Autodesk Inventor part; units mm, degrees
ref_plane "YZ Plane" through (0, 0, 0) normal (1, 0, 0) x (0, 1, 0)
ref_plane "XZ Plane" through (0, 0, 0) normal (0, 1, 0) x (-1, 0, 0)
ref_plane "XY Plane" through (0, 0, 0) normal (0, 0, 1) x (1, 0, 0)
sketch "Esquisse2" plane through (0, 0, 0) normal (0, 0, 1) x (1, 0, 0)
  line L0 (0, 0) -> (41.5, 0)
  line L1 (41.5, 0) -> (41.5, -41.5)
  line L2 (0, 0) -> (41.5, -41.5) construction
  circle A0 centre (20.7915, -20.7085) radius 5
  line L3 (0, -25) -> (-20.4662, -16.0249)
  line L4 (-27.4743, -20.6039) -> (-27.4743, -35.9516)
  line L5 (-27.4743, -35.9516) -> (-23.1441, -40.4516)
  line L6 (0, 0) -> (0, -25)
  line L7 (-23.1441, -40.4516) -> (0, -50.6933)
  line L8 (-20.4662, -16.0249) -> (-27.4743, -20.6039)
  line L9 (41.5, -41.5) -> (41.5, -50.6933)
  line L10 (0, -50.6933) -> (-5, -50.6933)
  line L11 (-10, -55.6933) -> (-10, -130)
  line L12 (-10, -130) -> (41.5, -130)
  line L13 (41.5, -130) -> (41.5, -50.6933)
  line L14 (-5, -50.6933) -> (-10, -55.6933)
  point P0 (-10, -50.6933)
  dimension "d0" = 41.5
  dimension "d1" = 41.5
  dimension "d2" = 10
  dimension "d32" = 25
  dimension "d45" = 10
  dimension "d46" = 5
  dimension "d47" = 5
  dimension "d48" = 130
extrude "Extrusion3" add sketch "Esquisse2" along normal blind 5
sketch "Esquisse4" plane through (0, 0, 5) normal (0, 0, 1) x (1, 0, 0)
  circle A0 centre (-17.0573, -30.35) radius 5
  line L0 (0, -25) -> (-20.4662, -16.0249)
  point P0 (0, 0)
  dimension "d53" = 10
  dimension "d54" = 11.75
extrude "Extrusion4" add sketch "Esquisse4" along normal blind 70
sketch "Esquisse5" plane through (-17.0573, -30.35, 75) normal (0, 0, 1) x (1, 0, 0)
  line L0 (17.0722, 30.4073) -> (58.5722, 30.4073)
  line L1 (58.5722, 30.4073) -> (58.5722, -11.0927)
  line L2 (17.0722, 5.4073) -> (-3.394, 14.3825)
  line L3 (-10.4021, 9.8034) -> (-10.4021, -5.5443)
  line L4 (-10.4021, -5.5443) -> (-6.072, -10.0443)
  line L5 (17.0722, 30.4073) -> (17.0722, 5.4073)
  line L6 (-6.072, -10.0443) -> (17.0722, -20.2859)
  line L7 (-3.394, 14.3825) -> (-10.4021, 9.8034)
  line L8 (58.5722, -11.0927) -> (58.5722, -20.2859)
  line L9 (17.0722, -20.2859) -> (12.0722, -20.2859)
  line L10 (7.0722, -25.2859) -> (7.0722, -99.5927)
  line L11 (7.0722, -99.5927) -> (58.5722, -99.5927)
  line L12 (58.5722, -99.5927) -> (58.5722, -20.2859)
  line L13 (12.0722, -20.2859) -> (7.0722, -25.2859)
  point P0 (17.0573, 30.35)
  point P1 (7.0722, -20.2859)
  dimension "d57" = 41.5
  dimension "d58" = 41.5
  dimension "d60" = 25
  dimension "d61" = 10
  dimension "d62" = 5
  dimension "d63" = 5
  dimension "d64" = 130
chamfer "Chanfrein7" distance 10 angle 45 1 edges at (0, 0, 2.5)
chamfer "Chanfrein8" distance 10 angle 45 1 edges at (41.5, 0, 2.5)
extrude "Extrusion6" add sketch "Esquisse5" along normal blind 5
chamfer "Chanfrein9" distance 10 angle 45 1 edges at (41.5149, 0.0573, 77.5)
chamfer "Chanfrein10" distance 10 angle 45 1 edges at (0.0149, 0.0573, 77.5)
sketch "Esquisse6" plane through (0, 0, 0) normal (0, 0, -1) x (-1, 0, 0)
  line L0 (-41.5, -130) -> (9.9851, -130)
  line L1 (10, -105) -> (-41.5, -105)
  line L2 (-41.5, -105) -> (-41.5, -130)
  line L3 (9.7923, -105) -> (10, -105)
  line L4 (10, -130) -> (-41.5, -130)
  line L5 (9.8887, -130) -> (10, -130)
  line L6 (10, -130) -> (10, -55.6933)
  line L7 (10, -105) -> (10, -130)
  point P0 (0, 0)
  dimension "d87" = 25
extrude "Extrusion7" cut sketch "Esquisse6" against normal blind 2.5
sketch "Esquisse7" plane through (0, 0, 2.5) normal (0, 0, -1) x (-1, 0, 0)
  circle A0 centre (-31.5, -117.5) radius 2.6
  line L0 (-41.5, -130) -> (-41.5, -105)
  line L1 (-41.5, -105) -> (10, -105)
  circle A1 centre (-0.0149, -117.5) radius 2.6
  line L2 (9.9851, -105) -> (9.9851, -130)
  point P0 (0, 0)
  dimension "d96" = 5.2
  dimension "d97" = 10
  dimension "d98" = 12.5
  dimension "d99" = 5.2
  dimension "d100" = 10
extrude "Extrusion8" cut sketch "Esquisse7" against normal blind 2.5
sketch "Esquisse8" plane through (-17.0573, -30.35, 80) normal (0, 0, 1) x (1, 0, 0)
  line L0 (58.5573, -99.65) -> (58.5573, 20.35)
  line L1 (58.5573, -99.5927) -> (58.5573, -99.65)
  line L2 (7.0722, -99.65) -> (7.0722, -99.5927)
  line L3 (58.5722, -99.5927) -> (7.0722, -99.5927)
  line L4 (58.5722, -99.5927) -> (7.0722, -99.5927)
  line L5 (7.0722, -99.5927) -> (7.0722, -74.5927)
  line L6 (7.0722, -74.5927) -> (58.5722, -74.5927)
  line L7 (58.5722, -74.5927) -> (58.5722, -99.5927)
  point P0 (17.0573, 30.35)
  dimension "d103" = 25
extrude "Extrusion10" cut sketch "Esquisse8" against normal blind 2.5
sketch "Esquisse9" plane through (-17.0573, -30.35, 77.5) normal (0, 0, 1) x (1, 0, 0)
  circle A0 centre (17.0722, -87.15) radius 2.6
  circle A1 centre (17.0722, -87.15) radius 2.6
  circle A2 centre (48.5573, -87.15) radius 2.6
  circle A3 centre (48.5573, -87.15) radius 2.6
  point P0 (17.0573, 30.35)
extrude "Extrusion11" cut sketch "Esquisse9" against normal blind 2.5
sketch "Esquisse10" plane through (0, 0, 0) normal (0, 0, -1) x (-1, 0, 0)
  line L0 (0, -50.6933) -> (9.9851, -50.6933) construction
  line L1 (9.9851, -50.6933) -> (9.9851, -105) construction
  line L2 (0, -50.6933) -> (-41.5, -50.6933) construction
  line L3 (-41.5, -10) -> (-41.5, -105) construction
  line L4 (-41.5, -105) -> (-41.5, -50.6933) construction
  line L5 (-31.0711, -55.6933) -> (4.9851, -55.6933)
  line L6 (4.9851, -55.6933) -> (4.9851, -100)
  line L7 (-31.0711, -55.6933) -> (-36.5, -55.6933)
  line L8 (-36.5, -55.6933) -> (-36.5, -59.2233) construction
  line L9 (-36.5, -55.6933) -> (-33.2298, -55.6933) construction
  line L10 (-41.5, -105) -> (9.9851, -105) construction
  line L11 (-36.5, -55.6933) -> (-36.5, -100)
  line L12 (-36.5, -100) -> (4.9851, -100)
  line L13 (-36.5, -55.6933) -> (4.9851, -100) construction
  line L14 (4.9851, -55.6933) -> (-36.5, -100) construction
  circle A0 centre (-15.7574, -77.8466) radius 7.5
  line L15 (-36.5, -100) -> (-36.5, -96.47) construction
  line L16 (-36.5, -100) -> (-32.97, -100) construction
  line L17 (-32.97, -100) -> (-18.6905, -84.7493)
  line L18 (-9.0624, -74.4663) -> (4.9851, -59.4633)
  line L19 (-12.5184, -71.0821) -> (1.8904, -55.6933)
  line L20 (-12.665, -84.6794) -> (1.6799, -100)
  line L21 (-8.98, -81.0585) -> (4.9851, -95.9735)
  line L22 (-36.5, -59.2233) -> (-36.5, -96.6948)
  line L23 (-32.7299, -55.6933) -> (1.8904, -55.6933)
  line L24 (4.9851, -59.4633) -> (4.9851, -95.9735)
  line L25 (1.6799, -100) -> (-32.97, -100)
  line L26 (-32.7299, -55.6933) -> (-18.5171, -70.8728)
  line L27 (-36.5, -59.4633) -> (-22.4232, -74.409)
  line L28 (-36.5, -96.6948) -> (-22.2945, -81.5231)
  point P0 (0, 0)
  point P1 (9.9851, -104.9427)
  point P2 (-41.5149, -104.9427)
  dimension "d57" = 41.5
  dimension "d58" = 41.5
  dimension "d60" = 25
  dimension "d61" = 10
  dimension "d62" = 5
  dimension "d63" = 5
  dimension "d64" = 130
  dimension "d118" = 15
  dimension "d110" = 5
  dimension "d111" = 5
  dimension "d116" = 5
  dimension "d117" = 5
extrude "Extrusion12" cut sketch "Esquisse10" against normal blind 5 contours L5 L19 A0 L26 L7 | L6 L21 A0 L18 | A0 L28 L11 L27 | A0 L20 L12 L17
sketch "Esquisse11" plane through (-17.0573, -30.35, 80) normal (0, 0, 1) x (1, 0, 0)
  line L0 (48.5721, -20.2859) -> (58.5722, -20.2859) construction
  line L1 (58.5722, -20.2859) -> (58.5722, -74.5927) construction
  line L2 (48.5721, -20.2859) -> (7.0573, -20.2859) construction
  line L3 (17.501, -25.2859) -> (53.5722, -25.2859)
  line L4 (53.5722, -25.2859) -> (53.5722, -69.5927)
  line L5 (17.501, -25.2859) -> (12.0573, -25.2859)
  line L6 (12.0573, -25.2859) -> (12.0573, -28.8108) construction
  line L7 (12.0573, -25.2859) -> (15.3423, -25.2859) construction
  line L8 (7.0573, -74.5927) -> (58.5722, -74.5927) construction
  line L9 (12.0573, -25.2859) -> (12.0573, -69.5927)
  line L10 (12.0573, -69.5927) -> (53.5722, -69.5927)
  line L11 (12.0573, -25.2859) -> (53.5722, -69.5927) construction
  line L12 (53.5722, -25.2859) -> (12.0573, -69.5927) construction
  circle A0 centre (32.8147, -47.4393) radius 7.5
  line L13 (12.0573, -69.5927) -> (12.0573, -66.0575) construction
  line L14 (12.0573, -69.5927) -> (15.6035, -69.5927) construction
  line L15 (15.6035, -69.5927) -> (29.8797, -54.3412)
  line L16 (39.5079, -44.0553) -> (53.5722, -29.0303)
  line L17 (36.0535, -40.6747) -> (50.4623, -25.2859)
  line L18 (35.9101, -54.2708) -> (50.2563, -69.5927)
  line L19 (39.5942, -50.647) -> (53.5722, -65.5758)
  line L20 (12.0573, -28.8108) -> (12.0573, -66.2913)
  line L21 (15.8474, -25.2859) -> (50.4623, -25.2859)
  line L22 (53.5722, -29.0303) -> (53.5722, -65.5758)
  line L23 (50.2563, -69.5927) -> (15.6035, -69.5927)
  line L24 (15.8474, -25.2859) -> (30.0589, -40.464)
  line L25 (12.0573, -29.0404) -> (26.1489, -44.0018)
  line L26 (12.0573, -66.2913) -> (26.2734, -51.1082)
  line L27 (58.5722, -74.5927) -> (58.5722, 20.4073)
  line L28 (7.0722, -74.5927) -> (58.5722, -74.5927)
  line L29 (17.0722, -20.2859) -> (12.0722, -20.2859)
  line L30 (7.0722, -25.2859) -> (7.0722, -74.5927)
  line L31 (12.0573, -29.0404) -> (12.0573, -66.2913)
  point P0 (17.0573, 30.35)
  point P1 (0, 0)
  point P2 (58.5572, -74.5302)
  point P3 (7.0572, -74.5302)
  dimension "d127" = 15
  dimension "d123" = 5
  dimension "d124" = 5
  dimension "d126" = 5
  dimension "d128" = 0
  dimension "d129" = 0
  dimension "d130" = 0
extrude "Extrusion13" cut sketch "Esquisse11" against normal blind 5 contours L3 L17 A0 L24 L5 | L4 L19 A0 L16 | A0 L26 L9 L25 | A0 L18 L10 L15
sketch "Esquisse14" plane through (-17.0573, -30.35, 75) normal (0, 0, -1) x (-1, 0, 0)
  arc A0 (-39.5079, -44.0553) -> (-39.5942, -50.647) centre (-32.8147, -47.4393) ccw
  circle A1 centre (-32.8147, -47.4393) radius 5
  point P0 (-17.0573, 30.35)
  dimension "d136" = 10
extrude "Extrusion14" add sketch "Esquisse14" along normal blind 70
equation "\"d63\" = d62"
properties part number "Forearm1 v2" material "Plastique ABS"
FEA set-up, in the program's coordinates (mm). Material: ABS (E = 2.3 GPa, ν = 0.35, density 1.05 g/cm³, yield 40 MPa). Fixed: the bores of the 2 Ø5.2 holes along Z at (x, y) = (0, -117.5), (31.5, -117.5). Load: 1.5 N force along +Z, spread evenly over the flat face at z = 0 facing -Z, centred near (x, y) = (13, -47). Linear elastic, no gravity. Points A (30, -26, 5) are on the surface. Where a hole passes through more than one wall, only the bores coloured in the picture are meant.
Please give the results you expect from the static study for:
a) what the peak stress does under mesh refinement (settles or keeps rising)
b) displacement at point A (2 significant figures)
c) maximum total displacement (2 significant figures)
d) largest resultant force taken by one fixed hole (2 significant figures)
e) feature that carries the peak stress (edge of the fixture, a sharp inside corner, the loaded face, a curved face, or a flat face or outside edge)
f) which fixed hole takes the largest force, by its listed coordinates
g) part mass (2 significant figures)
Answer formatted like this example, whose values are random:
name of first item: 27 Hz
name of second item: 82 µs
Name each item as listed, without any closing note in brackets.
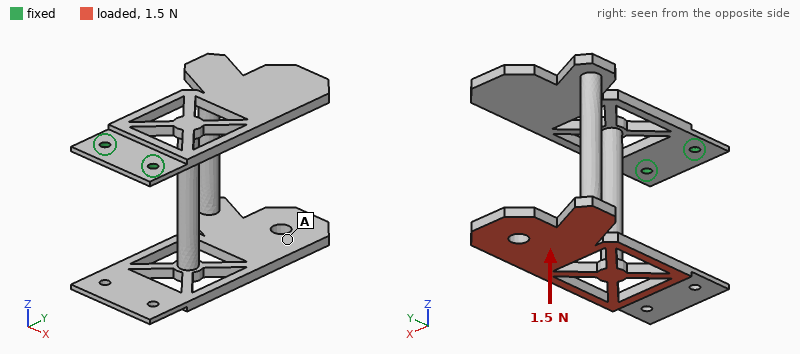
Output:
what the peak stress does under mesh refinement: keeps rising
displacement at point A: 1.4 mm
maximum total displacement: 1.7 mm
largest resultant force taken by one fixed hole: 0.84 N
feature that carries the peak stress: edge of the fixture
which fixed hole takes the largest force, by its listed coordinates: (0, -117.5)
part mass: 62 g
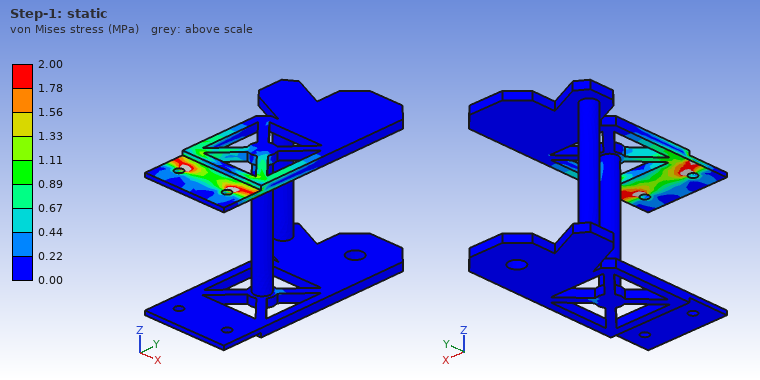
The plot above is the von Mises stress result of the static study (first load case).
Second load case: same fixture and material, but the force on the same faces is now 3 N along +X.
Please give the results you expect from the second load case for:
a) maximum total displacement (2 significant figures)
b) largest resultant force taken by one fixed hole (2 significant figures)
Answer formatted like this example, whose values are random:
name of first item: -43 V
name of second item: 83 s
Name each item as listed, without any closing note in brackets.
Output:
maximum total displacement: 1.7 mm
largest resultant force taken by one fixed hole: 8.6 N
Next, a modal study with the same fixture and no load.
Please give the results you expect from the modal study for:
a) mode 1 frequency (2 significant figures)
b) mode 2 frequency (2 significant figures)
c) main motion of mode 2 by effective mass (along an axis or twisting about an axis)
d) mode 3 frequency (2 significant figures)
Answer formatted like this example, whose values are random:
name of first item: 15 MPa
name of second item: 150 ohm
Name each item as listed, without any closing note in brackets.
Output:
mode 1 frequency: 21 Hz
mode 2 frequency: 42 Hz
main motion of mode 2 by effective mass: along X
mode 3 frequency: 120 Hz
